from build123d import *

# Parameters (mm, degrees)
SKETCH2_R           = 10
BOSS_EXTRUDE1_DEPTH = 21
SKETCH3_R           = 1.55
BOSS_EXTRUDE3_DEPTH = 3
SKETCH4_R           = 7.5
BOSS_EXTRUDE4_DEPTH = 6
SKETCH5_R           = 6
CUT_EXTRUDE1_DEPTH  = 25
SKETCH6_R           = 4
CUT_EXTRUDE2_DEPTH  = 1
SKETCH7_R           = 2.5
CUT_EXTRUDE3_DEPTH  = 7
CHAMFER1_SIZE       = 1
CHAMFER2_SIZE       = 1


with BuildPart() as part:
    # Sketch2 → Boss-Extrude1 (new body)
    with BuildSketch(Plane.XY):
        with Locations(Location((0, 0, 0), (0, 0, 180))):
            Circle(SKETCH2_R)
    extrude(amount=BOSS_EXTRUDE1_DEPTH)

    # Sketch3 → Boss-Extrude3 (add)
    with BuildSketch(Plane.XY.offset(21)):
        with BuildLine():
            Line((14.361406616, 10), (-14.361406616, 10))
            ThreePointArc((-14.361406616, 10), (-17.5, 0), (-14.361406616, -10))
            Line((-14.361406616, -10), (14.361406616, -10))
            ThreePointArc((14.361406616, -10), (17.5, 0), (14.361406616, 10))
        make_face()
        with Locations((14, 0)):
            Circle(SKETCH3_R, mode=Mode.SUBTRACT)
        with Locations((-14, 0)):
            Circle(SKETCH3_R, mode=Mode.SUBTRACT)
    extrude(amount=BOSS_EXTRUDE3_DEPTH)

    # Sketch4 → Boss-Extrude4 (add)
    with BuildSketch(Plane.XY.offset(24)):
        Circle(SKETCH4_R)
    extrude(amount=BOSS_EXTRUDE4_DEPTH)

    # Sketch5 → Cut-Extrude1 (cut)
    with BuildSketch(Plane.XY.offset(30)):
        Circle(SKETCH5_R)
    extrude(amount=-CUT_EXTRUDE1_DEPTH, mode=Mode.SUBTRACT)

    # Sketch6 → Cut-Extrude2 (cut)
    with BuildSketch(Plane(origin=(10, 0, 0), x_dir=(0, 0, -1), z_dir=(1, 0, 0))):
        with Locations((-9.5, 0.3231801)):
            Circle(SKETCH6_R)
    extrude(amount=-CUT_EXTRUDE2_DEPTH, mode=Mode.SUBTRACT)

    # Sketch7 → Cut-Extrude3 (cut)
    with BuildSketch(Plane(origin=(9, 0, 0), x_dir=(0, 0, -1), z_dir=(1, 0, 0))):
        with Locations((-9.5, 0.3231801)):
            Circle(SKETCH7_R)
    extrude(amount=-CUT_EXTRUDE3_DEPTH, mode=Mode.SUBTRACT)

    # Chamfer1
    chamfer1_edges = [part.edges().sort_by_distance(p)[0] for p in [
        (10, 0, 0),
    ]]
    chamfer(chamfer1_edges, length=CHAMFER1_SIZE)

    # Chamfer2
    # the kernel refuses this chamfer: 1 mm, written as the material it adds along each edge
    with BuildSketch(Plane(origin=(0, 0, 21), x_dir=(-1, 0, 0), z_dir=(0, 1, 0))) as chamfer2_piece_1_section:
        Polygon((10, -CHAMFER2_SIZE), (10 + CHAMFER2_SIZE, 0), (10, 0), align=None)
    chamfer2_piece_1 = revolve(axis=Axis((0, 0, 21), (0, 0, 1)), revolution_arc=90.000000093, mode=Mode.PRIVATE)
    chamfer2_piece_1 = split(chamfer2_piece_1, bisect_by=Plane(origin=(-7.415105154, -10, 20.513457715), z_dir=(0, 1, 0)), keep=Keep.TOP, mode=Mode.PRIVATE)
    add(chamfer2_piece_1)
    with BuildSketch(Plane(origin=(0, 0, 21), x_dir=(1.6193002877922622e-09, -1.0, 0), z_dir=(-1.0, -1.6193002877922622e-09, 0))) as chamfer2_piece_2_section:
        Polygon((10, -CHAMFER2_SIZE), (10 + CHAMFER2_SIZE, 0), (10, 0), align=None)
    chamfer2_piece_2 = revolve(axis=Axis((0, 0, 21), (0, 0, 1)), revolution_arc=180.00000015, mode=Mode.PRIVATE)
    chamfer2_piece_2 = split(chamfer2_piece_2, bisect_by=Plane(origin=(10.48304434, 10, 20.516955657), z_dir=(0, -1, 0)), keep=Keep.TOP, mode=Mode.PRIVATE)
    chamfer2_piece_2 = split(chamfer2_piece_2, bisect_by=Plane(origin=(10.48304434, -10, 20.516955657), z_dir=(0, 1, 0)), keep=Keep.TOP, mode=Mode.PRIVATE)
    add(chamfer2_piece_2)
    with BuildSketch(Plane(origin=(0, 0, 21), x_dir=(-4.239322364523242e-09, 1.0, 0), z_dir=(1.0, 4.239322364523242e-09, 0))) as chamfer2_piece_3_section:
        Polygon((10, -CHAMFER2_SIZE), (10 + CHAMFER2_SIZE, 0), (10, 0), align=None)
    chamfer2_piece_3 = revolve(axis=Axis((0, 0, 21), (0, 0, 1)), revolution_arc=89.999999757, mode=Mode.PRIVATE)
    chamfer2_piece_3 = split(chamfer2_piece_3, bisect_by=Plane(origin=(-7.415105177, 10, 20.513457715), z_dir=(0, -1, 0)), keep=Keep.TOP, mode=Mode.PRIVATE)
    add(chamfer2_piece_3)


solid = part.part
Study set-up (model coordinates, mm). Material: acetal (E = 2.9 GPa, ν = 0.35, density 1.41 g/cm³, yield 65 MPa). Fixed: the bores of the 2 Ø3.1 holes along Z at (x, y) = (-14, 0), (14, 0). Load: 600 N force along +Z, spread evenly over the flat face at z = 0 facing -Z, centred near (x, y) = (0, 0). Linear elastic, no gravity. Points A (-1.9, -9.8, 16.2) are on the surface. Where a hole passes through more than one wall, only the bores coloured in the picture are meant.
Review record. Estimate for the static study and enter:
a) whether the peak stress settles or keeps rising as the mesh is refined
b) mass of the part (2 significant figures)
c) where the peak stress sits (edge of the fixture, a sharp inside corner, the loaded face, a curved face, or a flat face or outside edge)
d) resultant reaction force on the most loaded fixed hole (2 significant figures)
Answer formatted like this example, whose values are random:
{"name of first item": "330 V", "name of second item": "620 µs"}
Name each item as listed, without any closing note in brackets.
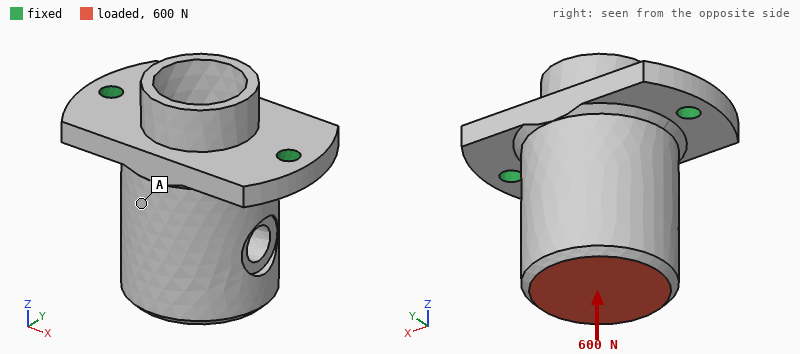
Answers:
{"whether the peak stress settles or keeps rising as the mesh is refined": "keeps rising", "mass of the part": "9.4 g", "where the peak stress sits": "edge of the fixture", "resultant reaction force on the most loaded fixed hole": "320 N"}
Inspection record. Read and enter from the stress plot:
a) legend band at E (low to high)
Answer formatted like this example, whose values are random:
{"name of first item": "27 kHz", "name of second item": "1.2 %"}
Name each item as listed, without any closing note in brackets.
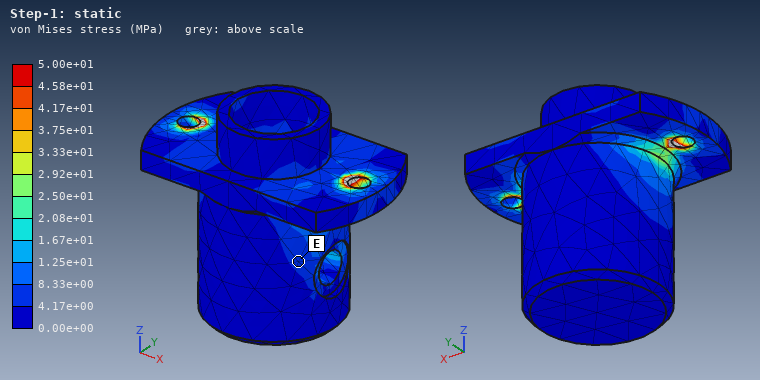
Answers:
{"legend band at E": "4.17e+00 to 8.33e+00 MPa"}
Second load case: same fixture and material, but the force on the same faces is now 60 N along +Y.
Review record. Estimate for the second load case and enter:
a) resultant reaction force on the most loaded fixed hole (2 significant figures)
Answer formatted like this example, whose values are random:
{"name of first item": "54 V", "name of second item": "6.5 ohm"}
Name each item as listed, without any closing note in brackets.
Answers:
{"resultant reaction force on the most loaded fixed hole": "30 N"}
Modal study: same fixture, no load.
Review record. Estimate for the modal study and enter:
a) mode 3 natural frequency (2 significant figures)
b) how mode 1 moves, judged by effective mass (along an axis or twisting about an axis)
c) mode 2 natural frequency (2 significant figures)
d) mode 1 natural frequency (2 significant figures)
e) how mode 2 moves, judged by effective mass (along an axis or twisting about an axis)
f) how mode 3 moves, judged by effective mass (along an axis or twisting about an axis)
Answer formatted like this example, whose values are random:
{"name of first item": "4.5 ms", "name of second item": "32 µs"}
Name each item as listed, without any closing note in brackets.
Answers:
{"mode 3 natural frequency": "4000 Hz", "how mode 1 moves, judged by effective mass": "along Y", "mode 2 natural frequency": "3200 Hz", "mode 1 natural frequency": "1000 Hz", "how mode 2 moves, judged by effective mass": "along X", "how mode 3 moves, judged by effective mass": "along Z"}
